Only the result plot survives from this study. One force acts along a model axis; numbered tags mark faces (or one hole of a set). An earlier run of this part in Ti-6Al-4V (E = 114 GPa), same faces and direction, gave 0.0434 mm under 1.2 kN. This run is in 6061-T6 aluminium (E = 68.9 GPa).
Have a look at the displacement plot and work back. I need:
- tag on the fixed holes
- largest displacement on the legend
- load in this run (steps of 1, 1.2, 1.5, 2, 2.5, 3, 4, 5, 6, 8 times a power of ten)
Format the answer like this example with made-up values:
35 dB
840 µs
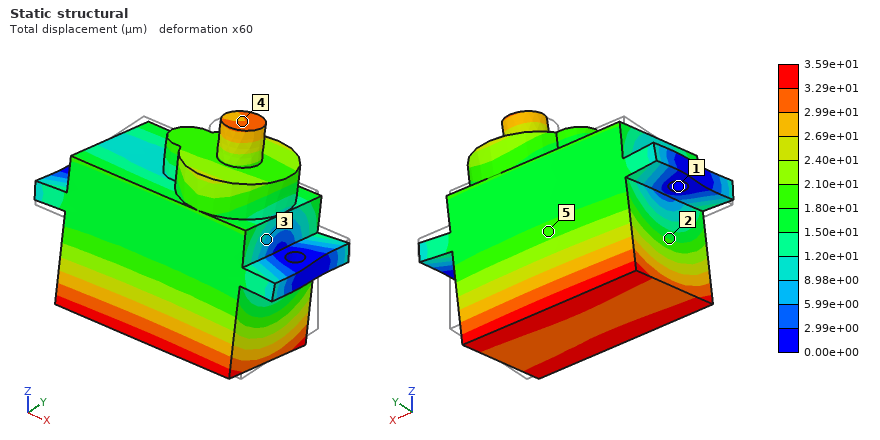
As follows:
1
3.59e+01 µm
600 N
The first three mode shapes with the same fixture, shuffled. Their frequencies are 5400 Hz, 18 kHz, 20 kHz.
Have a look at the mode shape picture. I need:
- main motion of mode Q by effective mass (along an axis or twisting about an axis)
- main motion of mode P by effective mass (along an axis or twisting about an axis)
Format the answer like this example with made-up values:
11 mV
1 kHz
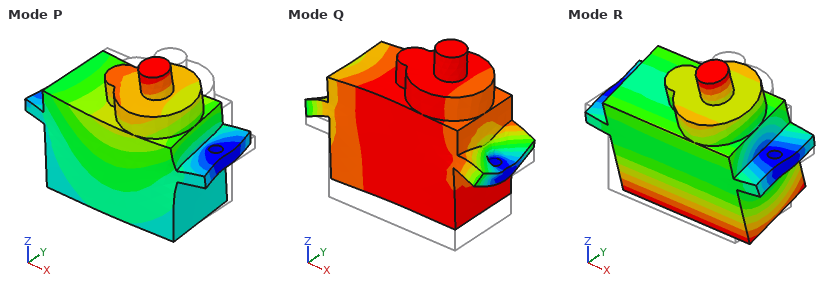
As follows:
along Z
along Y
